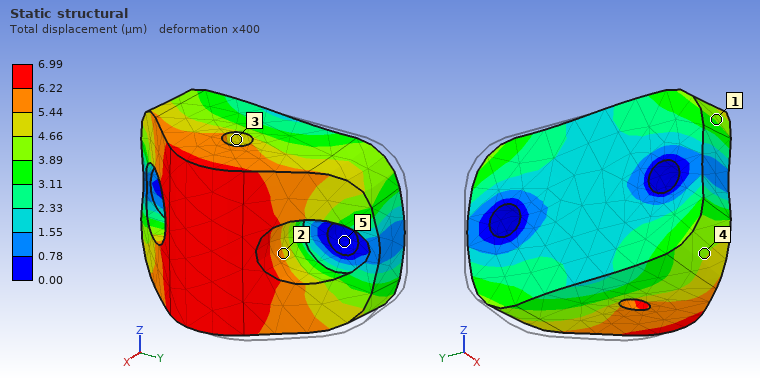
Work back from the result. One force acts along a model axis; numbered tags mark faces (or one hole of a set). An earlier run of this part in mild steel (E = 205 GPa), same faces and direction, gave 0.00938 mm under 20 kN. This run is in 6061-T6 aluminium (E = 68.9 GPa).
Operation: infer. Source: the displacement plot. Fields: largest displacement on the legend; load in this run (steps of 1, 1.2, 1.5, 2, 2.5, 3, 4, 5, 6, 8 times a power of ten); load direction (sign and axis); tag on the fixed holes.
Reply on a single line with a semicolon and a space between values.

6.99 µm; 5 kN; -Y; 5
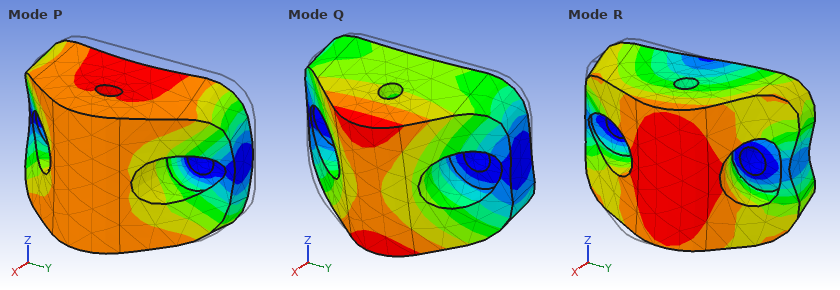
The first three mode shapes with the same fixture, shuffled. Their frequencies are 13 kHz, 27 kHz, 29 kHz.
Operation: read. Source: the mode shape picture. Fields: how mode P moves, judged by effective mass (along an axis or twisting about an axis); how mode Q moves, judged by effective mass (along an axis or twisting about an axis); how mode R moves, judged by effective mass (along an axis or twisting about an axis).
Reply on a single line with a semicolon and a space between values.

along X; along Z; along Y
